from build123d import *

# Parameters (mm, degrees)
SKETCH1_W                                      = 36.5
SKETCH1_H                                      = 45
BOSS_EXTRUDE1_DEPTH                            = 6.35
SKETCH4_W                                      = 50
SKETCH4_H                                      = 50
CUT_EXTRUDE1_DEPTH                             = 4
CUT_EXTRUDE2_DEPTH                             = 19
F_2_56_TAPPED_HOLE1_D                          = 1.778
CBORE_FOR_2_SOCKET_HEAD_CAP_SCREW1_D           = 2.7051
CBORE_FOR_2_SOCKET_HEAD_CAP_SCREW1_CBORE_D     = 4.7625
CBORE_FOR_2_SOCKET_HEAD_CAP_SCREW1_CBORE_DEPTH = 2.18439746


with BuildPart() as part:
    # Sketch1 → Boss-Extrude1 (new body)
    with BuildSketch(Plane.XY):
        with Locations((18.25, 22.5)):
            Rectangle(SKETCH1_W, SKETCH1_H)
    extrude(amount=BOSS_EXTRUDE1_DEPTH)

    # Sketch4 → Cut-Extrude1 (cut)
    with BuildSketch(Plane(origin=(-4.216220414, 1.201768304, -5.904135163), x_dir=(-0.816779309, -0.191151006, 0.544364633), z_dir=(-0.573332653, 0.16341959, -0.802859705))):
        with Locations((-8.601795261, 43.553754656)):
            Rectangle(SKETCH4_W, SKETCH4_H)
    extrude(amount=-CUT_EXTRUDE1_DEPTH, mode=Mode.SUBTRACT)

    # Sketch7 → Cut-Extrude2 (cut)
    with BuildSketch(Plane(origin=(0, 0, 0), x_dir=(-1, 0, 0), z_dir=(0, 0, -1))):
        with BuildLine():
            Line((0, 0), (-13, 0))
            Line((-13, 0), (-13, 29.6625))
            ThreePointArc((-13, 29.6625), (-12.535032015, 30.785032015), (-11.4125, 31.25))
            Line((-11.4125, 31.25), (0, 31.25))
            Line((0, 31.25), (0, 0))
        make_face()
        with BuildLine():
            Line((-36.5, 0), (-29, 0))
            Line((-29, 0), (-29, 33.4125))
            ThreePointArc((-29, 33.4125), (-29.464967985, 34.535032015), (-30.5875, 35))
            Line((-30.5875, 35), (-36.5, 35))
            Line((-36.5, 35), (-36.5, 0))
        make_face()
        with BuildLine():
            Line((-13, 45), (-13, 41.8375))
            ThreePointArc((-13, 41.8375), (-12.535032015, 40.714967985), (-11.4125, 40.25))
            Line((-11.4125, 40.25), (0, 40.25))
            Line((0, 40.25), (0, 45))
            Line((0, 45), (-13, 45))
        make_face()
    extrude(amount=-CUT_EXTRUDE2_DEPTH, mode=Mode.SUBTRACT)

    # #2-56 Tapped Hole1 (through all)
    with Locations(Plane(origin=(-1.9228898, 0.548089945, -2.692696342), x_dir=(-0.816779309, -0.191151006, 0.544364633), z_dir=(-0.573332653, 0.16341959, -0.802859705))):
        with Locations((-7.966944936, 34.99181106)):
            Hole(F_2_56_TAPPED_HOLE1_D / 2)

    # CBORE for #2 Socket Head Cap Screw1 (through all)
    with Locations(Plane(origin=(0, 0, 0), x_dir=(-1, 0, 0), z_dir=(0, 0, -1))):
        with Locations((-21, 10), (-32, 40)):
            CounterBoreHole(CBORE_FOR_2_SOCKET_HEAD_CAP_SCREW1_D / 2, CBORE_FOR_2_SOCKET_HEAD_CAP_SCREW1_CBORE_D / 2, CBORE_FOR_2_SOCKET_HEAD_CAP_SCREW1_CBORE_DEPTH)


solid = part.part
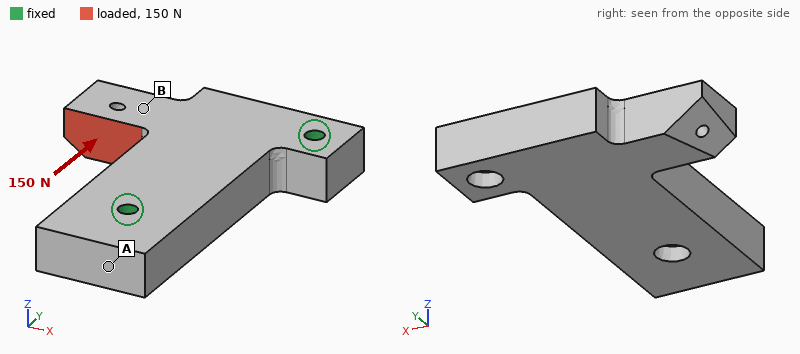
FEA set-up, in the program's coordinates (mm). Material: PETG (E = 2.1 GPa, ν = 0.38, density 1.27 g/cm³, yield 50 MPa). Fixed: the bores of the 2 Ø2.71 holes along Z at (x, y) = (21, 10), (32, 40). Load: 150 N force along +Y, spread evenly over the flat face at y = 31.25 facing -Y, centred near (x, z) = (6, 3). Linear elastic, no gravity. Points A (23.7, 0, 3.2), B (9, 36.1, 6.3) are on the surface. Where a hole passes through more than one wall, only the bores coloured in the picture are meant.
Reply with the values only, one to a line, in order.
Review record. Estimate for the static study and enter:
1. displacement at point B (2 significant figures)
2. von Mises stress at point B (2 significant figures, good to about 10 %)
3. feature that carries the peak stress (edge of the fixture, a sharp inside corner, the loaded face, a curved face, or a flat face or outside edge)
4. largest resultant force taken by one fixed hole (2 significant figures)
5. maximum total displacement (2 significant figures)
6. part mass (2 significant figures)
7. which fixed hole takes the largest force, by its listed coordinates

0.094 mm
6.1 MPa
a curved face
170 N
0.22 mm
7.1 g
(21, 10)
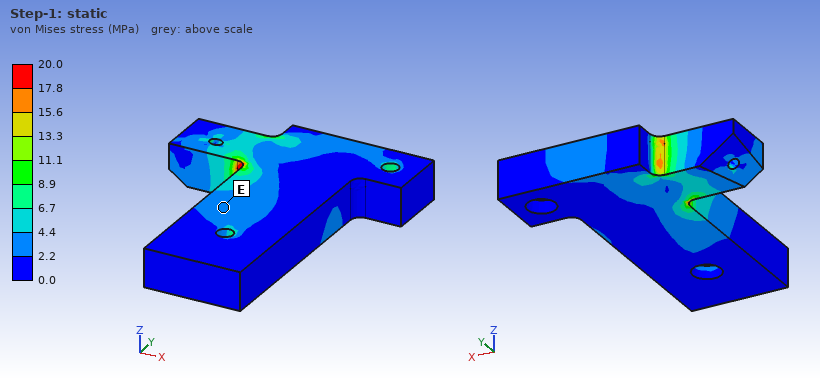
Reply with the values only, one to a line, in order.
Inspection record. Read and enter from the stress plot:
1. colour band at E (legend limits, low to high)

2.2 to 4.4 MPa
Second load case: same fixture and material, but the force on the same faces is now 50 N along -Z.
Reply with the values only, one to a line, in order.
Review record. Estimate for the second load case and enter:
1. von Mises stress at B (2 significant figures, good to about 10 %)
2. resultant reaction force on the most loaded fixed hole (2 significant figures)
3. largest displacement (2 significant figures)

4.1 MPa
28 N
0.62 mm
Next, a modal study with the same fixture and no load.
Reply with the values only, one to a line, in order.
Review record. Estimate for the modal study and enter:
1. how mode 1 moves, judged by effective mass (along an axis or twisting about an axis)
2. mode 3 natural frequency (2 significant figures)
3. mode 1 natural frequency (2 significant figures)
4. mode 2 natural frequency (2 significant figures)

along Z
5400 Hz
1600 Hz
4900 Hz
